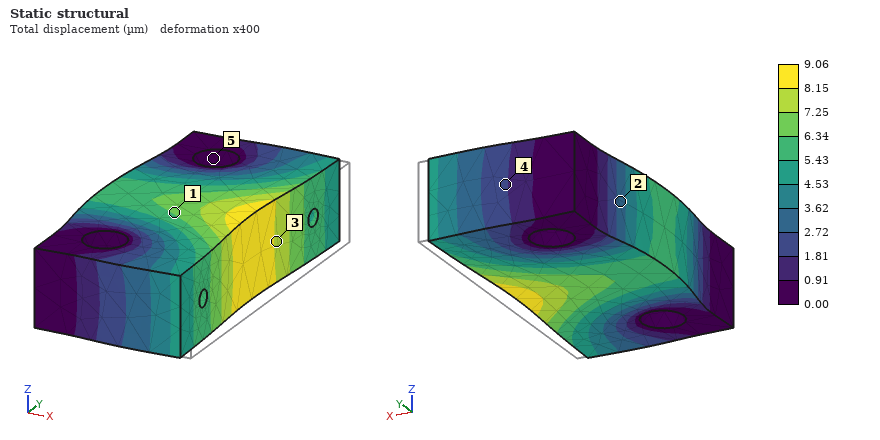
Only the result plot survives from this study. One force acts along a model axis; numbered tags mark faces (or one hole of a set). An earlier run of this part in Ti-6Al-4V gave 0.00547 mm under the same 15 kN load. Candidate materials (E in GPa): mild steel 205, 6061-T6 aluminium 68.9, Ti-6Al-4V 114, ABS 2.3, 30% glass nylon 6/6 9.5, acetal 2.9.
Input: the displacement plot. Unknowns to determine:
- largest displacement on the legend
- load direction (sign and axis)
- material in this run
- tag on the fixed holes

9.06 µm
-X
6061-T6 aluminium
5
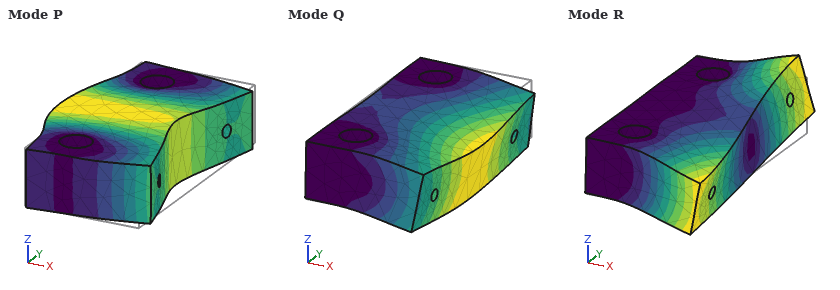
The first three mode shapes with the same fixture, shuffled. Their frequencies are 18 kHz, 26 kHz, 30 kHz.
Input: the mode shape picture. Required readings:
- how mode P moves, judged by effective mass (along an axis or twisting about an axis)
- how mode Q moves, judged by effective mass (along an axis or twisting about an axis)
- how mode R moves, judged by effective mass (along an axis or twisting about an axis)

along X
along Z
twisting about X
